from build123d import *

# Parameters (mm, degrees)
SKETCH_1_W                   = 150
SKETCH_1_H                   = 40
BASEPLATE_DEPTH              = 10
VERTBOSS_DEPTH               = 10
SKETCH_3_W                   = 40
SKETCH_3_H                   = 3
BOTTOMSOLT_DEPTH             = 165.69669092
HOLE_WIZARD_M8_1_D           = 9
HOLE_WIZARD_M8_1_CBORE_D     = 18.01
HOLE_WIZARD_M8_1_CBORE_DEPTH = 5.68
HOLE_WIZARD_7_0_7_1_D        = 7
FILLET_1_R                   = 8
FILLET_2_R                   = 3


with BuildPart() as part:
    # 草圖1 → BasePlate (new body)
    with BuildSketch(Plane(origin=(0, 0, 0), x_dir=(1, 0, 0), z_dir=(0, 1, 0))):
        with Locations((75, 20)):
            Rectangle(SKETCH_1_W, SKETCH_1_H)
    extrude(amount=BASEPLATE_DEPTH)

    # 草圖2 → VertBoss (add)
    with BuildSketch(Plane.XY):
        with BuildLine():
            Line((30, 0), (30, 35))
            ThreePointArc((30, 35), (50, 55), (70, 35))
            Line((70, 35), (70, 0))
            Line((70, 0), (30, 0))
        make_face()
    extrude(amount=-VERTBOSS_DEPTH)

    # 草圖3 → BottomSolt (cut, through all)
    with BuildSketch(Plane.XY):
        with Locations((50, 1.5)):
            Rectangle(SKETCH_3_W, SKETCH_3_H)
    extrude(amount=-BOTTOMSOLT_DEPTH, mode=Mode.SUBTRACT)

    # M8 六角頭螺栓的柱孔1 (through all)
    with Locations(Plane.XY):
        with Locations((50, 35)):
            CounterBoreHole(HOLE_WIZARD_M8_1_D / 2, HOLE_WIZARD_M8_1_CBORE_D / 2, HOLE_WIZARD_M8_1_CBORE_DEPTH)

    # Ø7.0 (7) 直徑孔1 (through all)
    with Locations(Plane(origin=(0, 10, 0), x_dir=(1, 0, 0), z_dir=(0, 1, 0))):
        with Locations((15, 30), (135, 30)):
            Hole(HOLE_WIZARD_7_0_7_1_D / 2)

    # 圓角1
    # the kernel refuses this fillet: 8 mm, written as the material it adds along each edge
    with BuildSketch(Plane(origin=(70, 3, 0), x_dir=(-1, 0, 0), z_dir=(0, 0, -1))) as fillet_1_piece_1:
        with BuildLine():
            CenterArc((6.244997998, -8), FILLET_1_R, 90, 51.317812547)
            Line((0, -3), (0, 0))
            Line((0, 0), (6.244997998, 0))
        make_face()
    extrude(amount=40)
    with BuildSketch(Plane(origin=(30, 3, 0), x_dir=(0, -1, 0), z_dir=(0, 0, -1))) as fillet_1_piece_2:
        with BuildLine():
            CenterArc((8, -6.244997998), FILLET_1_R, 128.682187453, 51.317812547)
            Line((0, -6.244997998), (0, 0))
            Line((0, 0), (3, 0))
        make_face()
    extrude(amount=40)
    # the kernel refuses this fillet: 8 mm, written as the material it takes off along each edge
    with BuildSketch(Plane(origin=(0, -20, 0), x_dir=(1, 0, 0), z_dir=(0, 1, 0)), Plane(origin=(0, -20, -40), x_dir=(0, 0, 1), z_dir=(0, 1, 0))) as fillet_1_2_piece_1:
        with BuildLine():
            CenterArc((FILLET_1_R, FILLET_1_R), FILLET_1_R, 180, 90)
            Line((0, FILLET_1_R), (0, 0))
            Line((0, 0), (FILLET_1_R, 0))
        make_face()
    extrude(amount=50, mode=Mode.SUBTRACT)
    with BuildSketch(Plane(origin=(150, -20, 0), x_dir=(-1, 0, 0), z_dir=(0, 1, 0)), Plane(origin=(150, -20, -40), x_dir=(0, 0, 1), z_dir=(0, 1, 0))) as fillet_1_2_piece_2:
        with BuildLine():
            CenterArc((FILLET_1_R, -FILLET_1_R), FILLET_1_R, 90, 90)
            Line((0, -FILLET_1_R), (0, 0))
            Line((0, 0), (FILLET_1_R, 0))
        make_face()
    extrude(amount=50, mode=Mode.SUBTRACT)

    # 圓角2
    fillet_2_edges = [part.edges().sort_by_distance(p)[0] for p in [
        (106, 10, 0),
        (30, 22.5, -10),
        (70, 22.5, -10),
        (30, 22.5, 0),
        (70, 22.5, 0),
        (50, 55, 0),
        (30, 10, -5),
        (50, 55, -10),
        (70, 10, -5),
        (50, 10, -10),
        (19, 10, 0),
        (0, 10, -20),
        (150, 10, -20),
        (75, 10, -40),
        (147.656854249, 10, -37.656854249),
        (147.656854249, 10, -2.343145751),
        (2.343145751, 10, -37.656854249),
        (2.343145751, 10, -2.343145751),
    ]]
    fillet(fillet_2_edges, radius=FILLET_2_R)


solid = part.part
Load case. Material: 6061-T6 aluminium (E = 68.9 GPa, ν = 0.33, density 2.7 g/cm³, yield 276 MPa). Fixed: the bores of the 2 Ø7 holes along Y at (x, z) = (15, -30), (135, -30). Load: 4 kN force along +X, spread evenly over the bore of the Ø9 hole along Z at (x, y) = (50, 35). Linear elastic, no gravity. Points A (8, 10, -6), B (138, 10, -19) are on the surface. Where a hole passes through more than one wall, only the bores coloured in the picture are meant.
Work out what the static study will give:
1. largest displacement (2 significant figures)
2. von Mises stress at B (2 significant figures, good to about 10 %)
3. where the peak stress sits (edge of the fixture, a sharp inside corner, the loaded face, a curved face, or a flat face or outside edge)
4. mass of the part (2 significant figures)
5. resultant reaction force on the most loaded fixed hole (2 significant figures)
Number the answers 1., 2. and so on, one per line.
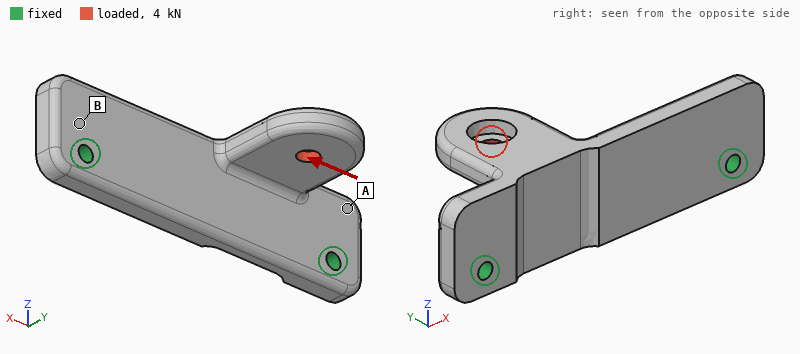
1. 0.30 mm
2. 32 MPa
3. a curved face
4. 180 g
5. 2.5 kN
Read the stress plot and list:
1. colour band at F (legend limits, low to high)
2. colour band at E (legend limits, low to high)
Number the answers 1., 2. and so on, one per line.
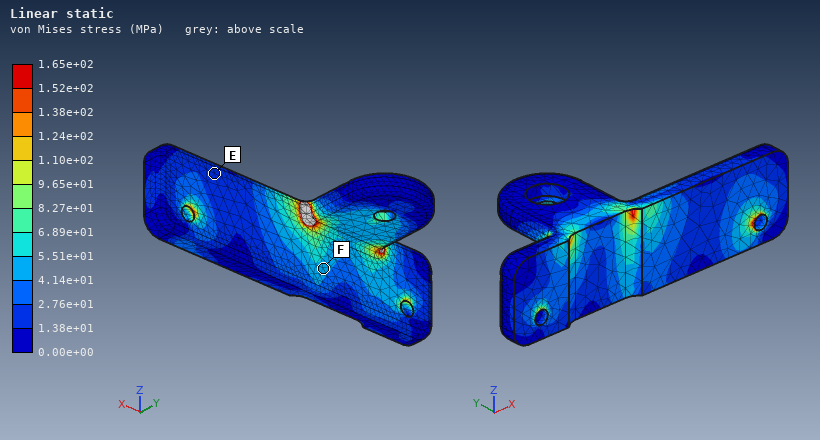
1. 4.14e+01 to 5.51e+01 MPa
2. 1.38e+01 to 2.76e+01 MPa
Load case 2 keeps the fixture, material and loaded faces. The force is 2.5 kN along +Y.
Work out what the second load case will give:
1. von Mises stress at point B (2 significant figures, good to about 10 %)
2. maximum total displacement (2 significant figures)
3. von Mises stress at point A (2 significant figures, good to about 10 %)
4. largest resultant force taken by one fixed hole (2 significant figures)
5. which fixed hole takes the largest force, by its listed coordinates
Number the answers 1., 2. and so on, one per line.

1. 24 MPa
2. 0.20 mm
3. 19 MPa
4. 1.9 kN
5. (15, -30)
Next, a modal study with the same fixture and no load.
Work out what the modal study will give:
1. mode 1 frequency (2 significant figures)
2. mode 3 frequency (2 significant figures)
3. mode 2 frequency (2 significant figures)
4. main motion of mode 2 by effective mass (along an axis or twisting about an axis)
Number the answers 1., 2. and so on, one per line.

1. 1900 Hz
2. 4900 Hz
3. 2600 Hz
4. along Y
